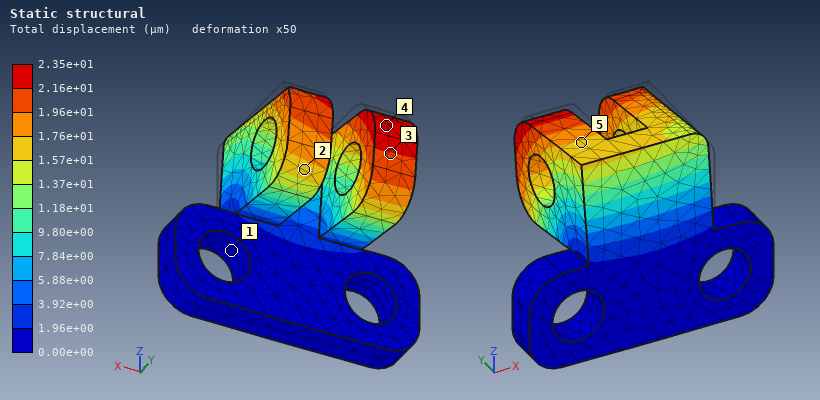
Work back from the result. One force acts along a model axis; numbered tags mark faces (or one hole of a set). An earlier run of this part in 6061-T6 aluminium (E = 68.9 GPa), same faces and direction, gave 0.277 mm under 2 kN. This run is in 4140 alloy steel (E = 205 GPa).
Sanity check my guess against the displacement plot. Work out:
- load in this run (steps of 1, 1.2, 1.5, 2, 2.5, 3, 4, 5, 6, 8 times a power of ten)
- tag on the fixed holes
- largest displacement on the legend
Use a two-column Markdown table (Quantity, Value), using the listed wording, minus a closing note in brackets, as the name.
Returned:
| Quantity | Value |
|---|---|
| load in this run | 500 N |
| tag on the fixed holes | 1 |
| largest displacement on the legend | 2.35e+01 µm |
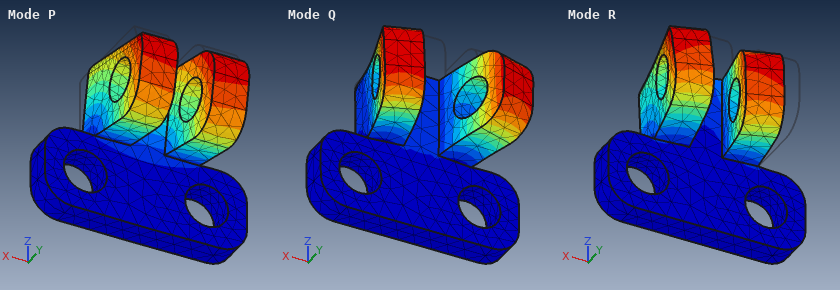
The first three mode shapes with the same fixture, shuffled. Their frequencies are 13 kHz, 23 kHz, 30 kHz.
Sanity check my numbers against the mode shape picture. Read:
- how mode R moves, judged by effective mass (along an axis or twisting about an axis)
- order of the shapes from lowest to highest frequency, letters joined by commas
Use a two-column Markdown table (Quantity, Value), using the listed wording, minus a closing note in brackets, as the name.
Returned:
| Quantity | Value |
|---|---|
| how mode R moves, judged by effective mass | along X |
| order of the shapes from lowest to highest frequency, letters joined by commas | P, R, Q |
